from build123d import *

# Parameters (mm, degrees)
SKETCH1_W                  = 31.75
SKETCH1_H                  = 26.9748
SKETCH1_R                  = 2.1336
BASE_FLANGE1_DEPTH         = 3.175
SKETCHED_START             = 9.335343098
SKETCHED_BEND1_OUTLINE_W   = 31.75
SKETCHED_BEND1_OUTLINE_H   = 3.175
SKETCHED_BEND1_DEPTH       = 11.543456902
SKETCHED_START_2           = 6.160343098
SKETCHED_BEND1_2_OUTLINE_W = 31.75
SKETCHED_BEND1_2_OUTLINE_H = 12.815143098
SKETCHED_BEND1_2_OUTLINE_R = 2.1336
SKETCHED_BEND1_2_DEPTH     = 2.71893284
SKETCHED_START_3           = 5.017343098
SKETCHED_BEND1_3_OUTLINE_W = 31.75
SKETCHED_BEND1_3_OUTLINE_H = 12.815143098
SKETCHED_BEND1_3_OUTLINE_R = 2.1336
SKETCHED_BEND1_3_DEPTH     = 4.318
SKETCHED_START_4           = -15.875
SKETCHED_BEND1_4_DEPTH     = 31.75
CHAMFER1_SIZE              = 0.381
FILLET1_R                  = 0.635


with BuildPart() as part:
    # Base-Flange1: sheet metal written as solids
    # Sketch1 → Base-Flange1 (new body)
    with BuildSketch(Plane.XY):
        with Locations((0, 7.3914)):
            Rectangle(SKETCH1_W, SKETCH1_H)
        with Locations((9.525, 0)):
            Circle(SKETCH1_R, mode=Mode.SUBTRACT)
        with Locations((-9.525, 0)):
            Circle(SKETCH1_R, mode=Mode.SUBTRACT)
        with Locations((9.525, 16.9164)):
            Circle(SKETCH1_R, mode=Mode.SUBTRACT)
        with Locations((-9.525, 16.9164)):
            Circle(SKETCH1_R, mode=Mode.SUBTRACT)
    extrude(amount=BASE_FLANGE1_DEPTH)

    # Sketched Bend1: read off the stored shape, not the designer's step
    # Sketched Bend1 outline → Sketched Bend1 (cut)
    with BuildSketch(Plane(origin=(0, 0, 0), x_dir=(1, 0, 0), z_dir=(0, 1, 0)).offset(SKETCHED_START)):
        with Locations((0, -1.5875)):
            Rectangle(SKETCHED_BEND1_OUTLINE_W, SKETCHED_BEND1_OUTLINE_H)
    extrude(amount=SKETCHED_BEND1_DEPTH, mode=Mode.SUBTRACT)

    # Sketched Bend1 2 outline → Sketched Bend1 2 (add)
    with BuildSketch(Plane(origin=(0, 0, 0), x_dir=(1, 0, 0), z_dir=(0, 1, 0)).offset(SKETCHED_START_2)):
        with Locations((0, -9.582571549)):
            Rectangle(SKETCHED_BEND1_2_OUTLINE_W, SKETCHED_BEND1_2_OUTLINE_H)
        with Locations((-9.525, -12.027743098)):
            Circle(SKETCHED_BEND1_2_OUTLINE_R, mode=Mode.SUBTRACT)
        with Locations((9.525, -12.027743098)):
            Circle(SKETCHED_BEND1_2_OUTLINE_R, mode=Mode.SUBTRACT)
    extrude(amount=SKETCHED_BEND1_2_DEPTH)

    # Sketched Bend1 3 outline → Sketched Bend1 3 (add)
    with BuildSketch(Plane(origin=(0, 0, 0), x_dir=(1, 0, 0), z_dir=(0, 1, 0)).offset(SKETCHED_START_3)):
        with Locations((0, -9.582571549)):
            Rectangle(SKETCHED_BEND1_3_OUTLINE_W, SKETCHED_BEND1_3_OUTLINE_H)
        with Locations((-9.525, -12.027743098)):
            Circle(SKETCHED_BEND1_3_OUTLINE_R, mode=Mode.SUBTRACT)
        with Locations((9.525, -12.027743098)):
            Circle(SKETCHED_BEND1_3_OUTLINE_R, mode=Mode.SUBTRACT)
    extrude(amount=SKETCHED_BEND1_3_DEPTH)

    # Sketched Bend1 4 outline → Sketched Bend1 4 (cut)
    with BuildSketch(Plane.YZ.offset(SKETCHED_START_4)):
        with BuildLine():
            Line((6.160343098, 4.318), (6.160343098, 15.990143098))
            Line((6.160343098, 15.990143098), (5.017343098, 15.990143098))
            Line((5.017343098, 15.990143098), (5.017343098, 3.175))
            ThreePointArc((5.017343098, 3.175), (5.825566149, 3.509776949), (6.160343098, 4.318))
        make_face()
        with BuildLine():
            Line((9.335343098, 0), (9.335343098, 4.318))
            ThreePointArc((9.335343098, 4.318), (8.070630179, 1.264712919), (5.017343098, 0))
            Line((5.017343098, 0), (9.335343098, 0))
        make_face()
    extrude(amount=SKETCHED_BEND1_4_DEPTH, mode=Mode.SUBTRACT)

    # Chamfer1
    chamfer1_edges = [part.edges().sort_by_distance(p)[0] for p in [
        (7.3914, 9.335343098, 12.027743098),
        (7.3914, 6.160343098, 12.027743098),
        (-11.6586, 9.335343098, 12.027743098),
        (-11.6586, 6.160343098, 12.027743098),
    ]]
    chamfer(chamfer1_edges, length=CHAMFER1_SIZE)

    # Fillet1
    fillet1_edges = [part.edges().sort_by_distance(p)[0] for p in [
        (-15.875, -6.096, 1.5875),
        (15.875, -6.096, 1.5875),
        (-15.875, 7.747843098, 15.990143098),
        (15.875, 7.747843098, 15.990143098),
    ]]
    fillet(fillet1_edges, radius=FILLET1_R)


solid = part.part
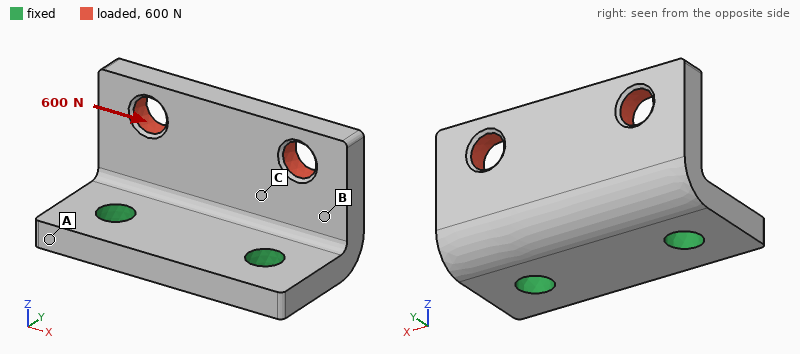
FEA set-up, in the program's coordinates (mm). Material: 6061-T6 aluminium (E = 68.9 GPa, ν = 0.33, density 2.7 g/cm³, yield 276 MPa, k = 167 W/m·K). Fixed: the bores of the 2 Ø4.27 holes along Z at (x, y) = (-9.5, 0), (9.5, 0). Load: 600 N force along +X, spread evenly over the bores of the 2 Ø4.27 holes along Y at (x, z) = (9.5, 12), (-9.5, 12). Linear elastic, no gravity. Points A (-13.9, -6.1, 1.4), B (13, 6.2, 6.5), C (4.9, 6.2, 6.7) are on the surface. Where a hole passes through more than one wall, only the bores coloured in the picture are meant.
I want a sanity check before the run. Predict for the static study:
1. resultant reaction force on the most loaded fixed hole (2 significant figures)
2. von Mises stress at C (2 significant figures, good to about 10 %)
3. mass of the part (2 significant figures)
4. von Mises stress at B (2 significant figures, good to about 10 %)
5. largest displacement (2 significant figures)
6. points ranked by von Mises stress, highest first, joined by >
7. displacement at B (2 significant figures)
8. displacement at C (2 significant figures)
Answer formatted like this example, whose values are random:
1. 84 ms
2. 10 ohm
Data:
1. 460 N
2. 28 MPa
3. 6.9 g
4. 21 MPa
5. 29 µm
6. C > B > A
7. 14 µm
8. 9.0 µm
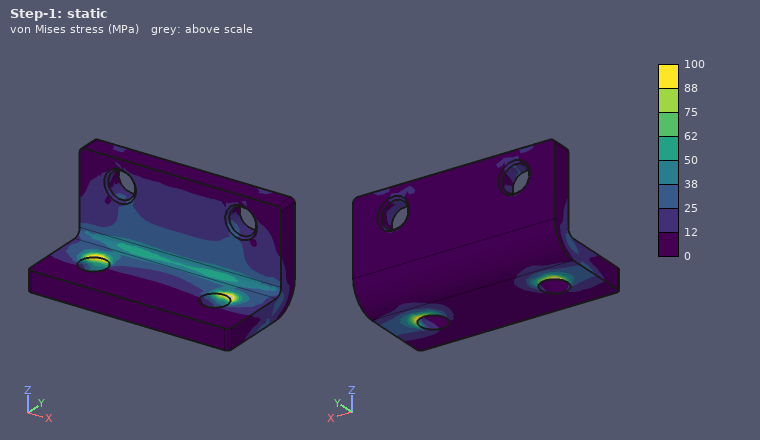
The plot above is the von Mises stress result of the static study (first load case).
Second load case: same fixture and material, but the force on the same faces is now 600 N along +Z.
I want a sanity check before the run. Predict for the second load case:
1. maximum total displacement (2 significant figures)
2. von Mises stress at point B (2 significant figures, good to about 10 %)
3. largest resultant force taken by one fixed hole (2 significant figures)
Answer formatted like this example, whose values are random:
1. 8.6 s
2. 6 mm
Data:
1. 43 µm
2. 9.2 MPa
3. 300 N
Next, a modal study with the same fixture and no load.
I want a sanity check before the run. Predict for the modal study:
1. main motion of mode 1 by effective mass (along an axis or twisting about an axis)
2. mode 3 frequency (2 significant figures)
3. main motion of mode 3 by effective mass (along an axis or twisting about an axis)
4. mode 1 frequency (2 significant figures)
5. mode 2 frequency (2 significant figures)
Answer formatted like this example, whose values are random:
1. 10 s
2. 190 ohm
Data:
1. along Y
2. 21 kHz
3. along X
4. 7700 Hz
5. 12 kHz
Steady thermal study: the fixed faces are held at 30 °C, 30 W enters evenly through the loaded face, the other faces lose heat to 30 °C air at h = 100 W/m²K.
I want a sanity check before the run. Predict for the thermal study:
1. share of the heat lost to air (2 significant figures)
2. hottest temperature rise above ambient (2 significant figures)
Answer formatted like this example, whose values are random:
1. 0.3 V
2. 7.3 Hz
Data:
1. 9.0 %
2. 35 K
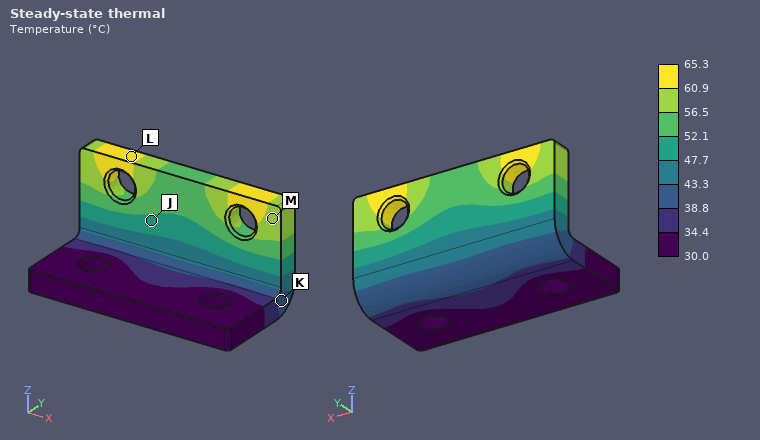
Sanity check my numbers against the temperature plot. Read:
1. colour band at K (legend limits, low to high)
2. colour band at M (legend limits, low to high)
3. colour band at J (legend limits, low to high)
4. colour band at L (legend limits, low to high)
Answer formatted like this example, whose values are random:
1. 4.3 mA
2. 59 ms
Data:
1. 38.8 to 43.3 °C
2. 56.5 to 60.9 °C
3. 47.7 to 52.1 °C
4. 60.9 to 65.3 °C
